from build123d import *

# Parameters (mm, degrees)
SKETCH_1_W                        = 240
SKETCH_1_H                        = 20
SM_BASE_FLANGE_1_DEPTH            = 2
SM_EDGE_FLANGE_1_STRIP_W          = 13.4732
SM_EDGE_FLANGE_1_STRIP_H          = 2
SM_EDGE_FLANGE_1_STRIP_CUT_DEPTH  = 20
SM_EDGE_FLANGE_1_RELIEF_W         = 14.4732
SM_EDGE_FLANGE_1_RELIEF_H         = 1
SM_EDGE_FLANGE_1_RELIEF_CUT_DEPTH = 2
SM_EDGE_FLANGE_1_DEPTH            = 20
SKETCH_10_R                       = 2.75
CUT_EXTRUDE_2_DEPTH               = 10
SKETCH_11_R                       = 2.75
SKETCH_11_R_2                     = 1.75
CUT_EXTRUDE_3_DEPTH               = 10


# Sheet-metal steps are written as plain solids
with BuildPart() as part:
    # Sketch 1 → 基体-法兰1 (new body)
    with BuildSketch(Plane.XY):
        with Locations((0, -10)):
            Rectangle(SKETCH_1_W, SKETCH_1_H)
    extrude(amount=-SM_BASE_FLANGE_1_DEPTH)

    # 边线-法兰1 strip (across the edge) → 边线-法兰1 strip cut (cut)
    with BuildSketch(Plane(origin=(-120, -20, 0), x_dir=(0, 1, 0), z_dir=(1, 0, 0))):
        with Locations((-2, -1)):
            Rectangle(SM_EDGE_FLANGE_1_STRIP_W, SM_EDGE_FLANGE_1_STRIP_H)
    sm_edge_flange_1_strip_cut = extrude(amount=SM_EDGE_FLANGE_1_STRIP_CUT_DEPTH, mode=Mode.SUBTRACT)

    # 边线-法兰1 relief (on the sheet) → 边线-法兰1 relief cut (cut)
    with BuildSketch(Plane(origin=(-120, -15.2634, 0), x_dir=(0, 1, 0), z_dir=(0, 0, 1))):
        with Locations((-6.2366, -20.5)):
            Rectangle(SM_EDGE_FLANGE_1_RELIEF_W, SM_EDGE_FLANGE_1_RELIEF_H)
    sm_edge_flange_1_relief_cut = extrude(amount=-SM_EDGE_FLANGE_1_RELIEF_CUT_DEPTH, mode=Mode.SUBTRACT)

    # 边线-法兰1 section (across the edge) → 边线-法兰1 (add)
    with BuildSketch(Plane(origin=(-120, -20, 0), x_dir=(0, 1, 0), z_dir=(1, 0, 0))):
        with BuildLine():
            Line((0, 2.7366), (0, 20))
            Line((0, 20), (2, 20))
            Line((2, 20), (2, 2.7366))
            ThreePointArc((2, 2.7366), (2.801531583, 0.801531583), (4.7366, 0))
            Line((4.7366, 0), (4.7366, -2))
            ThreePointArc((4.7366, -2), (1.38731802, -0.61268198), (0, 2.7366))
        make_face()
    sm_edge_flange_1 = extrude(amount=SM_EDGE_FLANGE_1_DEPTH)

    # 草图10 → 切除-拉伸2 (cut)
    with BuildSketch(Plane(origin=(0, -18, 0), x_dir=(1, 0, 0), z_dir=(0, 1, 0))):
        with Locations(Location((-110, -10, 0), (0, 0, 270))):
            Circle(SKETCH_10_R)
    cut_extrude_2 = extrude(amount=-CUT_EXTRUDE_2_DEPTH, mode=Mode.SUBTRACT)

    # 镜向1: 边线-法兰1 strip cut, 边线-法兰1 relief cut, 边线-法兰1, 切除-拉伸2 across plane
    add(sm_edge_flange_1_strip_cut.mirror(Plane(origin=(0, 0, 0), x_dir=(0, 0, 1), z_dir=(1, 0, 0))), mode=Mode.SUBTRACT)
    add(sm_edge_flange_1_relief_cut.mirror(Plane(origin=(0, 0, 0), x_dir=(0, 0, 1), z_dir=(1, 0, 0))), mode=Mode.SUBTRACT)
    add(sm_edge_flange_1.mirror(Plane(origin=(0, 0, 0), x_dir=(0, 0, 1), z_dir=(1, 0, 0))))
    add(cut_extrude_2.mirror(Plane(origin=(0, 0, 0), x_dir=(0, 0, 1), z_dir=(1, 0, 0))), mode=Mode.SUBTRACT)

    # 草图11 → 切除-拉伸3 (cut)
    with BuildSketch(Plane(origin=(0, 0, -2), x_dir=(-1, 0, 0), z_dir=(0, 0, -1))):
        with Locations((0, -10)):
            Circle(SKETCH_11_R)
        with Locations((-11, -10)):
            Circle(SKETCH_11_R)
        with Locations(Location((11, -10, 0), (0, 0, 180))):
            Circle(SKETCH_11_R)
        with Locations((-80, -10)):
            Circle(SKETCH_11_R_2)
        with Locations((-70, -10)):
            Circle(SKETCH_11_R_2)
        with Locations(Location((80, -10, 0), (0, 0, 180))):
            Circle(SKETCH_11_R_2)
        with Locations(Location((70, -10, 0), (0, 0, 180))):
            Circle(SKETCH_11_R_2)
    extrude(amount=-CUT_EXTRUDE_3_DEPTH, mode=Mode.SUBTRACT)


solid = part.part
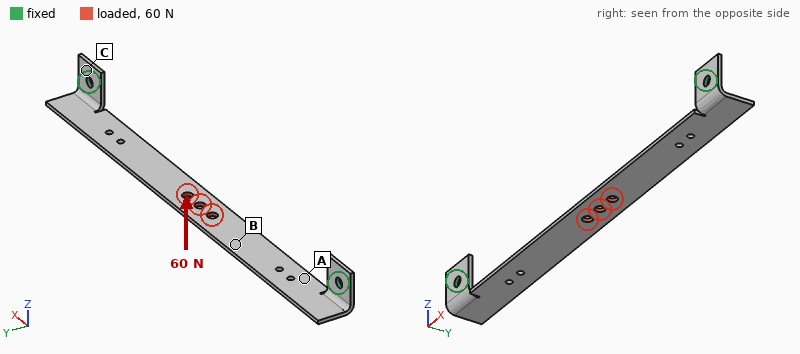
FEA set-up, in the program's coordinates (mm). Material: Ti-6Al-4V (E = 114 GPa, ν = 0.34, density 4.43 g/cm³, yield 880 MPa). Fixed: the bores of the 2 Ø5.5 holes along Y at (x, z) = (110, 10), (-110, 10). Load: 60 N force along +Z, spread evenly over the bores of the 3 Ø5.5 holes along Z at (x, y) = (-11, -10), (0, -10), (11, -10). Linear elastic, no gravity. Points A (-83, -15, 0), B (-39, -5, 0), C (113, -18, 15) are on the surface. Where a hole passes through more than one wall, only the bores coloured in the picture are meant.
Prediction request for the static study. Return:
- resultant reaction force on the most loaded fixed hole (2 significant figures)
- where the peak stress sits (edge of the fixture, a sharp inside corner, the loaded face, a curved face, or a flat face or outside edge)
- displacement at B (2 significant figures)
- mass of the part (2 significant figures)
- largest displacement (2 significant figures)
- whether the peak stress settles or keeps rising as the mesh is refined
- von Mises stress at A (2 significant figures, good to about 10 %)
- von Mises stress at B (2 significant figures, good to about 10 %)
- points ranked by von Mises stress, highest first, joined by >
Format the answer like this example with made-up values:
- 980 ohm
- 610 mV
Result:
- 30 N
- a sharp inside corner
- 1.7 mm
- 48 g
- 2.4 mm
- keeps rising
- 68 MPa
- 38 MPa
- A > B > C
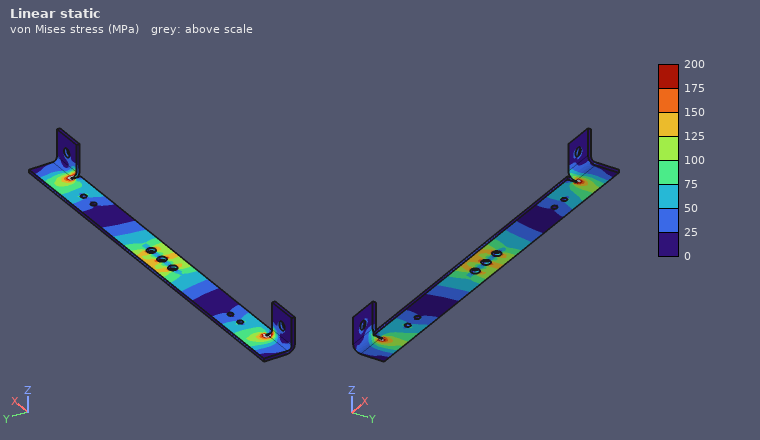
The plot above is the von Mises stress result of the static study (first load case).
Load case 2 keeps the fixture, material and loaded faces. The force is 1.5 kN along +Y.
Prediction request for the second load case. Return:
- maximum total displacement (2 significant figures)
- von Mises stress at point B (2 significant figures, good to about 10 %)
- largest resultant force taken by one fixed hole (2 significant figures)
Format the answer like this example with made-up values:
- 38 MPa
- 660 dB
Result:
- 1.8 mm
- 180 MPa
- 2.1 kN
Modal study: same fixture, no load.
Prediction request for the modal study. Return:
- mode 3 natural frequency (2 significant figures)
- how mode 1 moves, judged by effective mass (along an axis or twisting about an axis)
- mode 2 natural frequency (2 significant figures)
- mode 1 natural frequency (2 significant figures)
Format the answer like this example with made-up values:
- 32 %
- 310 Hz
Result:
- 970 Hz
- along Z
- 580 Hz
- 210 Hz
